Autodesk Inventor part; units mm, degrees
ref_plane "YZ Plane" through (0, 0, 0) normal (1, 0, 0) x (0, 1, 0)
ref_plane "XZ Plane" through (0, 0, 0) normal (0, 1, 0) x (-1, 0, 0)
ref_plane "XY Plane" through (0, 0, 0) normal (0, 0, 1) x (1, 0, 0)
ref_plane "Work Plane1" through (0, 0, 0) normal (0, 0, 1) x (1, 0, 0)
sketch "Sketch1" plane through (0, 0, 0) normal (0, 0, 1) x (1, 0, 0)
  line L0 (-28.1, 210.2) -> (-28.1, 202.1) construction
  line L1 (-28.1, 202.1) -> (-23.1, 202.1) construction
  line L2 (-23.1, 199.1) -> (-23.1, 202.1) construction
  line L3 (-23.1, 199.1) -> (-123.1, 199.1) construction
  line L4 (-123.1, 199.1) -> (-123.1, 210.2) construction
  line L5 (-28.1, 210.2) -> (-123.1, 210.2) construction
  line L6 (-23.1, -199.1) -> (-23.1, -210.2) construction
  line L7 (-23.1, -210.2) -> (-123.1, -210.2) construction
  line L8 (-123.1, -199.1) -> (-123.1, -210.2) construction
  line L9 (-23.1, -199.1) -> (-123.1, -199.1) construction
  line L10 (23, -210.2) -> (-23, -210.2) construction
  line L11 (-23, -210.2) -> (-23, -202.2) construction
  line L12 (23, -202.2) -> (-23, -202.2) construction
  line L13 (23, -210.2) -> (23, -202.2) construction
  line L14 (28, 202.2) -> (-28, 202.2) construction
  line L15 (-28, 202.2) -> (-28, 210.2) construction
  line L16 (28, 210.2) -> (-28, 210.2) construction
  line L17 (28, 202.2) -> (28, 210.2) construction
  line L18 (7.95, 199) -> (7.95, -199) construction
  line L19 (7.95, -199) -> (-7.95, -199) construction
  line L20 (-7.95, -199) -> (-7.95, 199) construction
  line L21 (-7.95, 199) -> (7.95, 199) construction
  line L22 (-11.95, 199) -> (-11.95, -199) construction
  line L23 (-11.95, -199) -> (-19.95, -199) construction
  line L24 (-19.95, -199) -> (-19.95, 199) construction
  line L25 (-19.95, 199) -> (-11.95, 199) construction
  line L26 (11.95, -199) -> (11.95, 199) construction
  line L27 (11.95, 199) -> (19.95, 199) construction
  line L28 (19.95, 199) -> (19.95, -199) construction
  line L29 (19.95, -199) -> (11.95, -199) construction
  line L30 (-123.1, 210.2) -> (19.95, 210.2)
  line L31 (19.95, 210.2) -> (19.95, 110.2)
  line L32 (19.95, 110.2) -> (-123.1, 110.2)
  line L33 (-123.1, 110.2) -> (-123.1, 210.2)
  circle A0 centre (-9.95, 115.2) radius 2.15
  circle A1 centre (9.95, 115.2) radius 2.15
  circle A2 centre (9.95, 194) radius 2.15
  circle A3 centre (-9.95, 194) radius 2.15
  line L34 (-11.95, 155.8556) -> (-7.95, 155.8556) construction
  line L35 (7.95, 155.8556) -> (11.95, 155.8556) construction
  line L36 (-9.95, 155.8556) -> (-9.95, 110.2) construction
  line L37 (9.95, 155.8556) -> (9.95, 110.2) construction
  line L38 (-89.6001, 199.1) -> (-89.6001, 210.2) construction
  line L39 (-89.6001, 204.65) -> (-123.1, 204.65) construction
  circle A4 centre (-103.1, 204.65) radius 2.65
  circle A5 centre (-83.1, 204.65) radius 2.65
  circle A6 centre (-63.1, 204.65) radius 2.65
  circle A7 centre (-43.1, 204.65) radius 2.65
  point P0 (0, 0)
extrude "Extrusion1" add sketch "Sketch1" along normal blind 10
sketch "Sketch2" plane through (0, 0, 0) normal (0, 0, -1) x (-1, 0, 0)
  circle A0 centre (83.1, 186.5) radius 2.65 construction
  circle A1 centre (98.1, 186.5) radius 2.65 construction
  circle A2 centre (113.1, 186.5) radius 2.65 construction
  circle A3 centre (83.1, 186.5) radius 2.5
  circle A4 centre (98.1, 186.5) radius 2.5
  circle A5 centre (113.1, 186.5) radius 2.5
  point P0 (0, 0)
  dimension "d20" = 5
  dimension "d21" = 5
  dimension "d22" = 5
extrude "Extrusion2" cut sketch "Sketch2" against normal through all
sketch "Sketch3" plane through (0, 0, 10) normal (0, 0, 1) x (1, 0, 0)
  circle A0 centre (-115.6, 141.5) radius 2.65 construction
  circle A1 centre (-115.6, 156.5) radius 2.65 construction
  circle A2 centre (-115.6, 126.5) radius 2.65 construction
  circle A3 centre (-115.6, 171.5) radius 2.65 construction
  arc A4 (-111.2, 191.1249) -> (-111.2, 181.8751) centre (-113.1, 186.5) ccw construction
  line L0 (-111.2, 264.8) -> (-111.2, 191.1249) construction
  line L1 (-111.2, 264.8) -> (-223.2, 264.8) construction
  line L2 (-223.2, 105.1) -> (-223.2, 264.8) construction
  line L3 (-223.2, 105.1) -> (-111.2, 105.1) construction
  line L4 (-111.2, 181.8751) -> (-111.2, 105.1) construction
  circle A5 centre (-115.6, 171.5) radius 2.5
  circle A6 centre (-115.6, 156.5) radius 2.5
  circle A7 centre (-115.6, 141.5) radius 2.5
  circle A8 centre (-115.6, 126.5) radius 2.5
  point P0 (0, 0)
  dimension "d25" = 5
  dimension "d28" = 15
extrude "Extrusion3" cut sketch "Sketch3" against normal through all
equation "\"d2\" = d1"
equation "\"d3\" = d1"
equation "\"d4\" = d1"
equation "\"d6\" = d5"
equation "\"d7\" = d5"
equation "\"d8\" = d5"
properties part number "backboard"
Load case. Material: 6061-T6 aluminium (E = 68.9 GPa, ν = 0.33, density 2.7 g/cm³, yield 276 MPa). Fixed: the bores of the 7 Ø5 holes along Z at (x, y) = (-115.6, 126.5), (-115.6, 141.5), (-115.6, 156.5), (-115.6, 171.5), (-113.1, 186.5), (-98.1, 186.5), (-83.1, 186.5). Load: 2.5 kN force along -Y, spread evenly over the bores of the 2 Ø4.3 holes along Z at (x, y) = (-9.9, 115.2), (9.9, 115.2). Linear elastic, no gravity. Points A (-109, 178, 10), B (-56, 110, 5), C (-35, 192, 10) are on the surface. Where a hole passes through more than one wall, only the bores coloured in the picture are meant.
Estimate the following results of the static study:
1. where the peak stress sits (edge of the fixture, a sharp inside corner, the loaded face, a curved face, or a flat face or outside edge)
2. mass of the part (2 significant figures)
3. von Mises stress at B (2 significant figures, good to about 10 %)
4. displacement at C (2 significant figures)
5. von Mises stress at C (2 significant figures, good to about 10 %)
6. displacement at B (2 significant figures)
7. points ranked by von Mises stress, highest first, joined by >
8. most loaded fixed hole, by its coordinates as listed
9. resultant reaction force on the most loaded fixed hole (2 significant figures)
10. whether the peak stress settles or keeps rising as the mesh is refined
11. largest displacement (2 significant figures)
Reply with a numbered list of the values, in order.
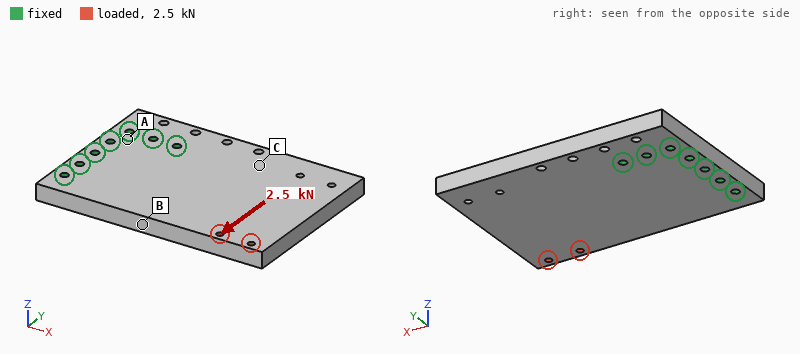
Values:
1. edge of the fixture
2. 380 g
3. 9.9 MPa
4. 18 µm
5. 4.8 MPa
6. 17 µm
7. B > C > A
8. (-83.1, 186.5)
9. 3.4 kN
10. keeps rising
11. 42 µm
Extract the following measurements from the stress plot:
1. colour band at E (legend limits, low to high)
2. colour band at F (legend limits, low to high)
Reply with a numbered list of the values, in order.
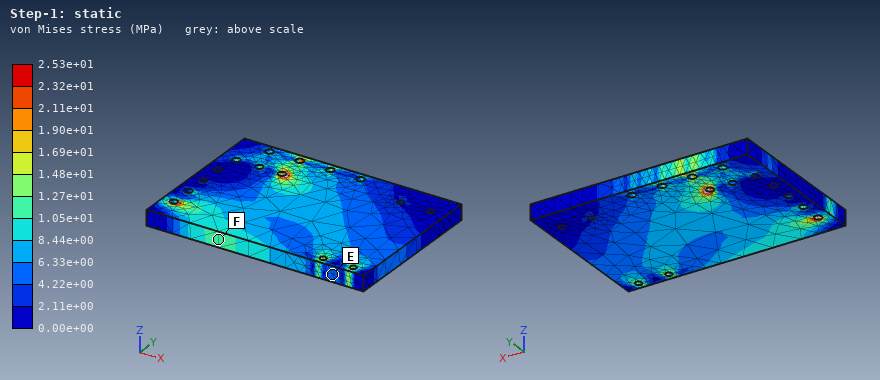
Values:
1. 4.22e+00 to 6.33e+00 MPa
2. 1.05e+01 to 1.27e+01 MPa
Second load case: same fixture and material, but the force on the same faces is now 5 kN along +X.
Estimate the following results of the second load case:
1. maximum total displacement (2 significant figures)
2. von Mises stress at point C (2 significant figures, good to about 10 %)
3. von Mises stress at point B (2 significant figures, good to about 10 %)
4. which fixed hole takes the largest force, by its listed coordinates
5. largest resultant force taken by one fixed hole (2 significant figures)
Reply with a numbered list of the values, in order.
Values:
1. 59 µm
2. 4.0 MPa
3. 20 MPa
4. (-115.6, 126.5)
5. 3.4 kN
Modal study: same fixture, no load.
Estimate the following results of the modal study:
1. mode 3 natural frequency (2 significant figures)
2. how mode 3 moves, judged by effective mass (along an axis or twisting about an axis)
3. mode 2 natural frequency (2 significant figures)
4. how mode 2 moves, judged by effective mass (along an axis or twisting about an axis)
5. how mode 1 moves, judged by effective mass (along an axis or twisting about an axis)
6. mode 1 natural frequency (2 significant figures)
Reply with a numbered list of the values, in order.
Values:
1. 3400 Hz
2. along Z
3. 1500 Hz
4. twisting about X
5. along Z
6. 620 Hz
